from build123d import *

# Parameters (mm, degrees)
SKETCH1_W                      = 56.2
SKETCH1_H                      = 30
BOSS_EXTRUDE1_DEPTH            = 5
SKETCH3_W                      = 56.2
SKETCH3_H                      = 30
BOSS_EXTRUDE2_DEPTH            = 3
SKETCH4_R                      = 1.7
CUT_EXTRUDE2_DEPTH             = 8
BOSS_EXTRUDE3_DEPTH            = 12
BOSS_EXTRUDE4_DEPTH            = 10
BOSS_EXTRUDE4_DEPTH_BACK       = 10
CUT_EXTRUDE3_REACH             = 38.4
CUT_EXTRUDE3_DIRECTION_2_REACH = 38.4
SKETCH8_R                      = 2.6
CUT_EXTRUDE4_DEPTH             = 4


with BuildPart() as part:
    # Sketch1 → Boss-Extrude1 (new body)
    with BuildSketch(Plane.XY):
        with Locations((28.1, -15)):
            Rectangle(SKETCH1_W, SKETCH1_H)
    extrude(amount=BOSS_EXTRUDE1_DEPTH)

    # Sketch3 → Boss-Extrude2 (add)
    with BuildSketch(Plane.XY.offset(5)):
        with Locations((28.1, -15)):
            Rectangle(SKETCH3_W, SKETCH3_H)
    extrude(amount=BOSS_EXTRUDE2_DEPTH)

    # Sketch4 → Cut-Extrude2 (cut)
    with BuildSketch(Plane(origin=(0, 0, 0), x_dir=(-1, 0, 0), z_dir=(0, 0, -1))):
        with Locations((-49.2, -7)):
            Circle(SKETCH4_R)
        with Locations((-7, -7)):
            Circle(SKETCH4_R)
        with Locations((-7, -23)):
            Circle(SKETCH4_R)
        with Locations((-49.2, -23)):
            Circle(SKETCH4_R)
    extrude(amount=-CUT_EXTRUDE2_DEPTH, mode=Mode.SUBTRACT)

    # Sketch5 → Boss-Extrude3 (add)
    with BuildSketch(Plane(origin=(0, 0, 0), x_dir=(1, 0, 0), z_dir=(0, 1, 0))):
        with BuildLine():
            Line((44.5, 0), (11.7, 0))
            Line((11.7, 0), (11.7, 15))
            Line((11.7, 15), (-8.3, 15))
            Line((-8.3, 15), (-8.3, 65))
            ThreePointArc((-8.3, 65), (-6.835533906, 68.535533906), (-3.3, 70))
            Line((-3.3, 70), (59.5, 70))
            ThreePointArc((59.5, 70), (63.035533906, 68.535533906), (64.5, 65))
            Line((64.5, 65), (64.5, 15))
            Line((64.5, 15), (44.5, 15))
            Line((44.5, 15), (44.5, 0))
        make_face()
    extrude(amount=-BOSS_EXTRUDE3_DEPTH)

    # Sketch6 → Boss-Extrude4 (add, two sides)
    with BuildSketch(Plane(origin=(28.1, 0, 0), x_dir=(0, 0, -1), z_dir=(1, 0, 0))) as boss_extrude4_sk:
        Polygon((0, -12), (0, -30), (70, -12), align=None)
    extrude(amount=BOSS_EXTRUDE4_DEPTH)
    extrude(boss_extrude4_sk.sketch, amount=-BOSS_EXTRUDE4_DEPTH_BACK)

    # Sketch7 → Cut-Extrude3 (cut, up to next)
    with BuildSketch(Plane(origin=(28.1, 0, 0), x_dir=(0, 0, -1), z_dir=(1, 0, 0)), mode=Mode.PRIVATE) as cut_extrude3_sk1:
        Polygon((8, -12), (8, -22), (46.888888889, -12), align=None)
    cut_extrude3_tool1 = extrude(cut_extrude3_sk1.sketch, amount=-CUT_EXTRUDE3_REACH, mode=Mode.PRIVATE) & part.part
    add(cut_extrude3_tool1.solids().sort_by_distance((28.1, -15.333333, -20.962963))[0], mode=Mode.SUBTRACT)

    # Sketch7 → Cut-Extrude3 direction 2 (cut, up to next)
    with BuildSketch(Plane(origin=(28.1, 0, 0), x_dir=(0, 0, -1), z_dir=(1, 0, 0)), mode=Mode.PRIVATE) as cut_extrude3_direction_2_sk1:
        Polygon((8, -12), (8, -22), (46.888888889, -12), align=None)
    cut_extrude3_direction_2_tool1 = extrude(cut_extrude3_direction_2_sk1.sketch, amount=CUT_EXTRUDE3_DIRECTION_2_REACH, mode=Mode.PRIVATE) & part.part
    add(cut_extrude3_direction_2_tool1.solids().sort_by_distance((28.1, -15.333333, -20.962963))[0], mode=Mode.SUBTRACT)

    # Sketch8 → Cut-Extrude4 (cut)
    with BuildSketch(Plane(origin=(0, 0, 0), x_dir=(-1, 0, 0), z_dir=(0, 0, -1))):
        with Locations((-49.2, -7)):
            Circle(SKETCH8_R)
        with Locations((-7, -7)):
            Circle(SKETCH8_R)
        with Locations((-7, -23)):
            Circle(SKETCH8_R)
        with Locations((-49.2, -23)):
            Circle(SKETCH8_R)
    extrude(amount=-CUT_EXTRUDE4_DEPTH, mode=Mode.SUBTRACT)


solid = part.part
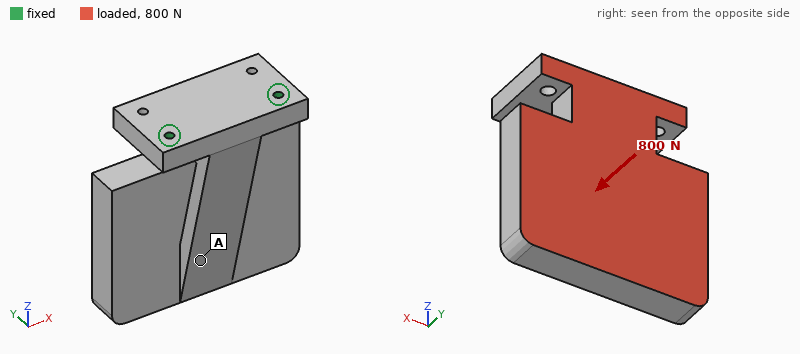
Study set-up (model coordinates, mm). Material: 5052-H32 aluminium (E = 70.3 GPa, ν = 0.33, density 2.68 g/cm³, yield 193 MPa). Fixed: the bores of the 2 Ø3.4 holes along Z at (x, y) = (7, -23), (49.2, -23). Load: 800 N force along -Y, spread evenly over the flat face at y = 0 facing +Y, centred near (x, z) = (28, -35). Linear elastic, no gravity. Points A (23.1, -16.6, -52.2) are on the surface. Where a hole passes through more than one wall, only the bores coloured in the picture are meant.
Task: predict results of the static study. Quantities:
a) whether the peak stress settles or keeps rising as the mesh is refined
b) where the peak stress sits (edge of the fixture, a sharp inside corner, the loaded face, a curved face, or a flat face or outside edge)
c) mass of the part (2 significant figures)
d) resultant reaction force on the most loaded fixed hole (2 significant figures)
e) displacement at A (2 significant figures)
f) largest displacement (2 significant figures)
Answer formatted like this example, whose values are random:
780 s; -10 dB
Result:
keeps rising; edge of the fixture; 200 g; 600 N; 0.37 mm; 0.51 mm
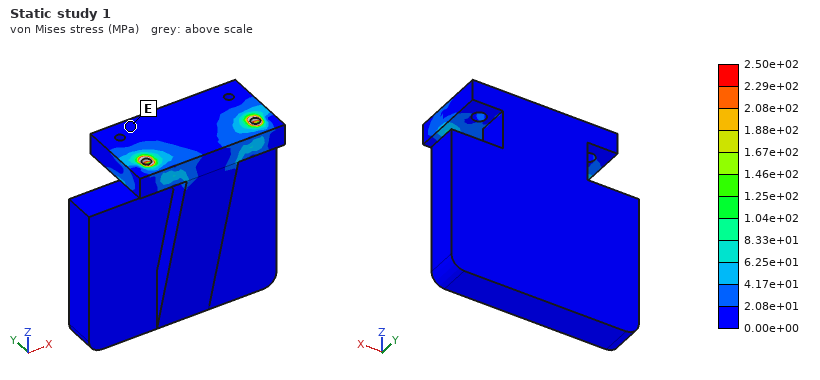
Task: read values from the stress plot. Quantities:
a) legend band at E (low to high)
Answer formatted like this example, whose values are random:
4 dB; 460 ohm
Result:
0.00e+00 to 2.08e+01 MPa
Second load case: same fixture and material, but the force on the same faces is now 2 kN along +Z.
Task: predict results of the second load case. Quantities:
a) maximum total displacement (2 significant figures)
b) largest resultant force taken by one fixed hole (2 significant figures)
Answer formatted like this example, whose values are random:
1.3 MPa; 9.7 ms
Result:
0.67 mm; 1.0 kN
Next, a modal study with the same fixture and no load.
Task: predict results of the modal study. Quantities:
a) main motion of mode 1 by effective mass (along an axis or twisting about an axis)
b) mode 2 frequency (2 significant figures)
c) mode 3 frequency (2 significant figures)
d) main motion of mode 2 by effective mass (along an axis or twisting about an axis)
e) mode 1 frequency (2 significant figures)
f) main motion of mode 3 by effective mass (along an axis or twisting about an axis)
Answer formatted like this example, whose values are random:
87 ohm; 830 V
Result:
along Y; 1600 Hz; 2900 Hz; along X; 560 Hz; twisting about Z
